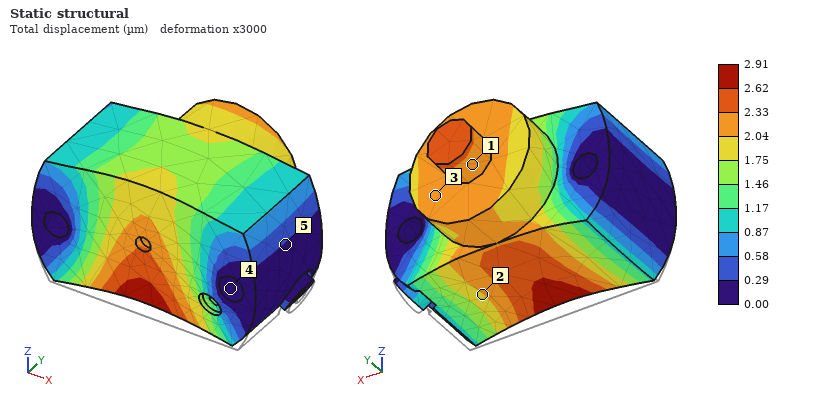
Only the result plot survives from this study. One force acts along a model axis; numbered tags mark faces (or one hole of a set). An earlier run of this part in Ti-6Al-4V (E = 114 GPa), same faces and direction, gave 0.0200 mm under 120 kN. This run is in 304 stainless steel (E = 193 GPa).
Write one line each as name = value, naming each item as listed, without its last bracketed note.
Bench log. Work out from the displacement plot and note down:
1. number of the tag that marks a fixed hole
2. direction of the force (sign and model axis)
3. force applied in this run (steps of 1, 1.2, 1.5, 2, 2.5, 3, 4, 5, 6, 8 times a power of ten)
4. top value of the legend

number of the tag that marks a fixed hole = 4
direction of the force = +Z
force applied in this run = 30 kN
top value of the legend = 2.91 µm
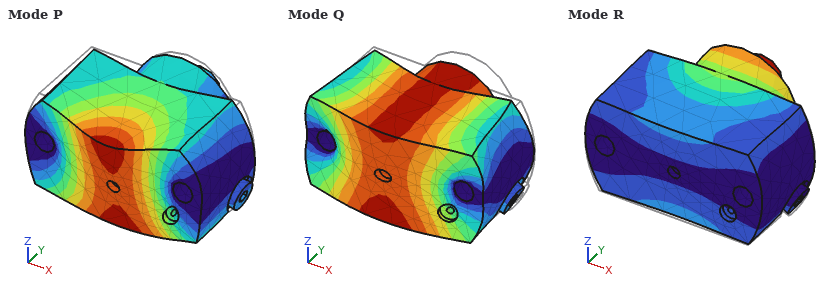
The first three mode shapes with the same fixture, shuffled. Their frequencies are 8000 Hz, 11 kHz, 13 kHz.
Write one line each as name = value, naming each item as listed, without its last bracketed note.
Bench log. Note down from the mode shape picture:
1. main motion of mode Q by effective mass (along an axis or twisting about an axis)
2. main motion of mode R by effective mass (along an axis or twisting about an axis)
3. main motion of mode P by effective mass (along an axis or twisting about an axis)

main motion of mode Q by effective mass = along Y
main motion of mode R by effective mass = along Z
main motion of mode P by effective mass = along Z
